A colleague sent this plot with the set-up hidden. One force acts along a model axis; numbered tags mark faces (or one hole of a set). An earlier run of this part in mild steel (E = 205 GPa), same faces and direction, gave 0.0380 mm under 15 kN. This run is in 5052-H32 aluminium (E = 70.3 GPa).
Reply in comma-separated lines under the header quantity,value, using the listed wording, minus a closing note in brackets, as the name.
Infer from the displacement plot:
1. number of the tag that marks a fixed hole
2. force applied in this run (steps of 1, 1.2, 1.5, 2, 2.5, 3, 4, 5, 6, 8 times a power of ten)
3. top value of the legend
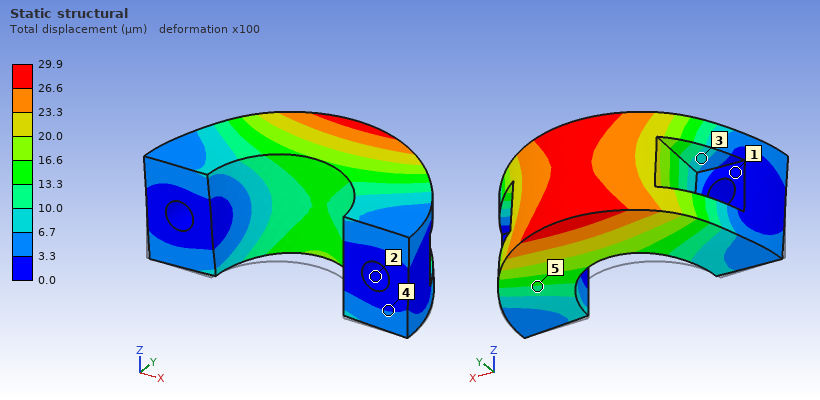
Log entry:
quantity,value
number of the tag that marks a fixed hole,2
force applied in this run,4 kN
top value of the legend,29.9 µm
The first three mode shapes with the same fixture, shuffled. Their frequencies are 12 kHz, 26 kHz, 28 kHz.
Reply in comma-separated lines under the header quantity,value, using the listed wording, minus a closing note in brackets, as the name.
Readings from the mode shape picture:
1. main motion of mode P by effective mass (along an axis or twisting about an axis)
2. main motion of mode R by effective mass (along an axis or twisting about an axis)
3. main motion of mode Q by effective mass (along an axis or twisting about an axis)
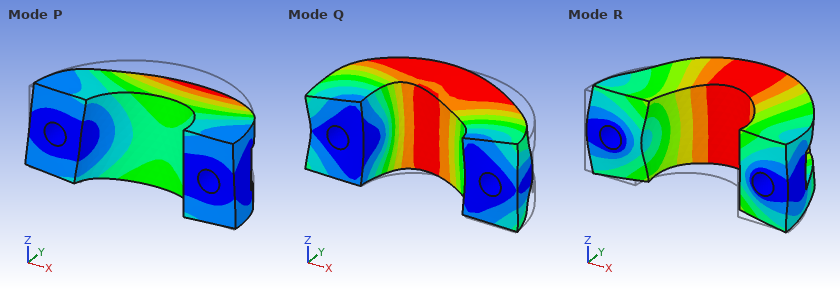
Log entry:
quantity,value
main motion of mode P by effective mass,along Z
main motion of mode R by effective mass,along Y
main motion of mode Q by effective mass,along X
